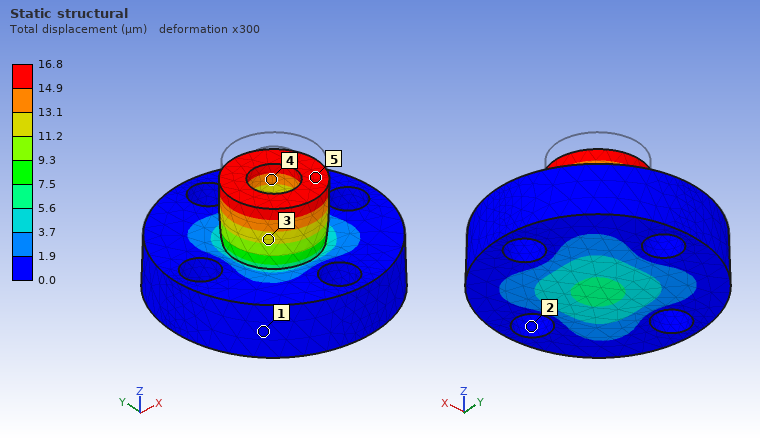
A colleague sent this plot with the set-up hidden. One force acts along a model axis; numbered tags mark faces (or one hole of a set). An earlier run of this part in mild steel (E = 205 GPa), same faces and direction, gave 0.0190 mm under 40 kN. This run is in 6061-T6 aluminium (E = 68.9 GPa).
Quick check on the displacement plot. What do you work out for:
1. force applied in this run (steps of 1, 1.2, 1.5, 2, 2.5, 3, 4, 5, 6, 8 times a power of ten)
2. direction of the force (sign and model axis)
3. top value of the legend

12 kN
-Z
16.8 µm
